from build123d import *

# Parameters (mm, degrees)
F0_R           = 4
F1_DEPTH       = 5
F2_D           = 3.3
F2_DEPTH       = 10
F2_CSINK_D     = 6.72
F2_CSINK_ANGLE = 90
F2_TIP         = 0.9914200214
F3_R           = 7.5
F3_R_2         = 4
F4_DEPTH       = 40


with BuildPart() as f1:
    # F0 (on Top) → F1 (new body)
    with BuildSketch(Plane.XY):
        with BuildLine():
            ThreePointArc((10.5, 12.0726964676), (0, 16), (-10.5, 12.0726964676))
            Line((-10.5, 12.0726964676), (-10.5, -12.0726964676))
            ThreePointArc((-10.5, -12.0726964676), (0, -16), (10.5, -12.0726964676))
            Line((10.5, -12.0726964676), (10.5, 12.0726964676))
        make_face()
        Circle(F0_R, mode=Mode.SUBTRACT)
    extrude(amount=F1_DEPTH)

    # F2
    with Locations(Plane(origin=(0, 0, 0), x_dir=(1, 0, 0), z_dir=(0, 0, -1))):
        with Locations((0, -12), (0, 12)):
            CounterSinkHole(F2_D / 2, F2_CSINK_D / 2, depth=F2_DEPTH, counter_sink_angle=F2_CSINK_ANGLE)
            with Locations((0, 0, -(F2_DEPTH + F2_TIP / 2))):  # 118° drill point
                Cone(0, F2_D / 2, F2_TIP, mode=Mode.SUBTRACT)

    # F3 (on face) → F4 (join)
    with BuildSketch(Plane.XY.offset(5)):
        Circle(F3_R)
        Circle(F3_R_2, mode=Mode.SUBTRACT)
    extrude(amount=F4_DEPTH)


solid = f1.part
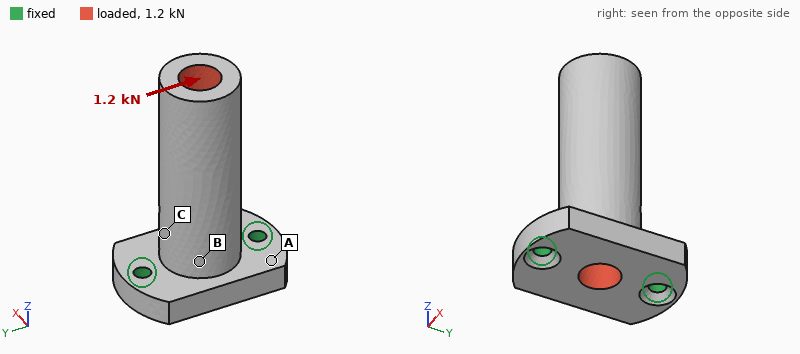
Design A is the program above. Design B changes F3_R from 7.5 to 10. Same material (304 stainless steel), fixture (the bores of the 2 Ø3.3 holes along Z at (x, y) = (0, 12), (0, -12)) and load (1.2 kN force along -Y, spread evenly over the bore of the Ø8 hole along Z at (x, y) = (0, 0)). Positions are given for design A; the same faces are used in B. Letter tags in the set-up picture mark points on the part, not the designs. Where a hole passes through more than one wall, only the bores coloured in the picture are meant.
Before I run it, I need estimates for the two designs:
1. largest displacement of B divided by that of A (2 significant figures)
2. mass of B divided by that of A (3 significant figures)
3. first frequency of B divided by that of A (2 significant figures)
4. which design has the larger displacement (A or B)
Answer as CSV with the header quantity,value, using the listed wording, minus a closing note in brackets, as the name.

quantity,value
largest displacement of B divided by that of A,0.33
mass of B divided by that of A,1.71
first frequency of B divided by that of A,0.84
which design has the larger displacement,A
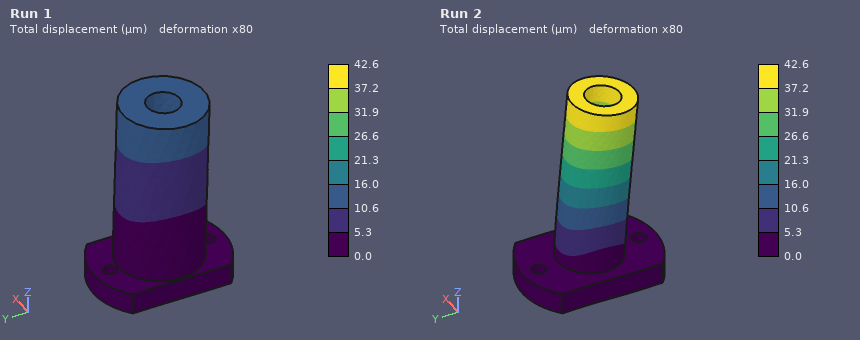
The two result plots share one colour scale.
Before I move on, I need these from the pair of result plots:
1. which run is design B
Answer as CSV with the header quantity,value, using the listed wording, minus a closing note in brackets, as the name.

quantity,value
which run is design B,Run 1
